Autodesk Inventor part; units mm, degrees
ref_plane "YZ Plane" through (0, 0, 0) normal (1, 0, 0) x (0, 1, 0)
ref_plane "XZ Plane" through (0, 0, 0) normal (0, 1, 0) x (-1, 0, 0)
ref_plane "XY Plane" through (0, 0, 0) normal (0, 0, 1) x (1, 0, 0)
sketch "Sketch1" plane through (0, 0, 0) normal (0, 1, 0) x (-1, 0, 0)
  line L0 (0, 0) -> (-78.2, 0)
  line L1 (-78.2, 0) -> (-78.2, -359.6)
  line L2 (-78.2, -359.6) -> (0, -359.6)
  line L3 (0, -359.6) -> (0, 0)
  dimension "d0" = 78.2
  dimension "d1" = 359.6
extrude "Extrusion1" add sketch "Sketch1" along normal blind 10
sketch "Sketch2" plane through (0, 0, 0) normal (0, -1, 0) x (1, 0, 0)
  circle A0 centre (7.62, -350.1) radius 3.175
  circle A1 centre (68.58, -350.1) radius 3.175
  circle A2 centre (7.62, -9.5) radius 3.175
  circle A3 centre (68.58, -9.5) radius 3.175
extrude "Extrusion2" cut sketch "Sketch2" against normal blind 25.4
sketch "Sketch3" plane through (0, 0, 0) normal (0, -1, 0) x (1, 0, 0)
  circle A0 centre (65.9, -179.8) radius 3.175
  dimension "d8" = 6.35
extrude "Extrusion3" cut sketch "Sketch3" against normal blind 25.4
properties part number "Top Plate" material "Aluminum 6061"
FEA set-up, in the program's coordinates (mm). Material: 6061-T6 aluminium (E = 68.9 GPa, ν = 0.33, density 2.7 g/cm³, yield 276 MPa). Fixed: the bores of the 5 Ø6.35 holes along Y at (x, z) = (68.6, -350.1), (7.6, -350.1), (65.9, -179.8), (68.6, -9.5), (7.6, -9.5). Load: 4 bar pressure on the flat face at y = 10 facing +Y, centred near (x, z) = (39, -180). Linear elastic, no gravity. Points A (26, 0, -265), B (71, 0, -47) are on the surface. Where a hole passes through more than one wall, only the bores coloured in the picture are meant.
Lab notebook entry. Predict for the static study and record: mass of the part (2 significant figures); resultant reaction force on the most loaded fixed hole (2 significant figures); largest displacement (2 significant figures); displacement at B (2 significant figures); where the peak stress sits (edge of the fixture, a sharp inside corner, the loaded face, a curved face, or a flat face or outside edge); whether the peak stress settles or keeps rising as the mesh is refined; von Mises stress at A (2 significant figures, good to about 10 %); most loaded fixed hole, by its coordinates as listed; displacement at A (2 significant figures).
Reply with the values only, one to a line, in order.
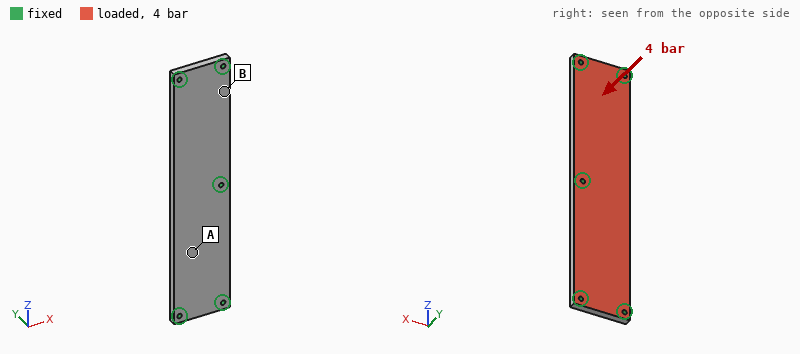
750 g
5.3 kN
0.37 mm
0.080 mm
edge of the fixture
keeps rising
32 MPa
(65.9, -179.8)
0.26 mm
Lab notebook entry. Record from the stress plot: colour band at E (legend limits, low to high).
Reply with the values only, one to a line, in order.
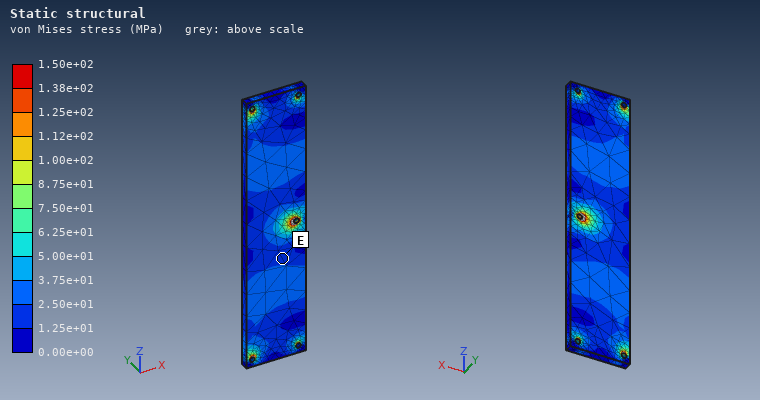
1.25e+01 to 2.50e+01 MPa
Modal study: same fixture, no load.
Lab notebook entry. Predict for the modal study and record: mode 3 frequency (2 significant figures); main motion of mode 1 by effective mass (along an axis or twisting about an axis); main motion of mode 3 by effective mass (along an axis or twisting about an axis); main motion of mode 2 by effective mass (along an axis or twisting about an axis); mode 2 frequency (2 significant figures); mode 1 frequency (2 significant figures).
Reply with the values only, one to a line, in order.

2100 Hz
along Y
along Y
twisting about X
1400 Hz
1300 Hz
